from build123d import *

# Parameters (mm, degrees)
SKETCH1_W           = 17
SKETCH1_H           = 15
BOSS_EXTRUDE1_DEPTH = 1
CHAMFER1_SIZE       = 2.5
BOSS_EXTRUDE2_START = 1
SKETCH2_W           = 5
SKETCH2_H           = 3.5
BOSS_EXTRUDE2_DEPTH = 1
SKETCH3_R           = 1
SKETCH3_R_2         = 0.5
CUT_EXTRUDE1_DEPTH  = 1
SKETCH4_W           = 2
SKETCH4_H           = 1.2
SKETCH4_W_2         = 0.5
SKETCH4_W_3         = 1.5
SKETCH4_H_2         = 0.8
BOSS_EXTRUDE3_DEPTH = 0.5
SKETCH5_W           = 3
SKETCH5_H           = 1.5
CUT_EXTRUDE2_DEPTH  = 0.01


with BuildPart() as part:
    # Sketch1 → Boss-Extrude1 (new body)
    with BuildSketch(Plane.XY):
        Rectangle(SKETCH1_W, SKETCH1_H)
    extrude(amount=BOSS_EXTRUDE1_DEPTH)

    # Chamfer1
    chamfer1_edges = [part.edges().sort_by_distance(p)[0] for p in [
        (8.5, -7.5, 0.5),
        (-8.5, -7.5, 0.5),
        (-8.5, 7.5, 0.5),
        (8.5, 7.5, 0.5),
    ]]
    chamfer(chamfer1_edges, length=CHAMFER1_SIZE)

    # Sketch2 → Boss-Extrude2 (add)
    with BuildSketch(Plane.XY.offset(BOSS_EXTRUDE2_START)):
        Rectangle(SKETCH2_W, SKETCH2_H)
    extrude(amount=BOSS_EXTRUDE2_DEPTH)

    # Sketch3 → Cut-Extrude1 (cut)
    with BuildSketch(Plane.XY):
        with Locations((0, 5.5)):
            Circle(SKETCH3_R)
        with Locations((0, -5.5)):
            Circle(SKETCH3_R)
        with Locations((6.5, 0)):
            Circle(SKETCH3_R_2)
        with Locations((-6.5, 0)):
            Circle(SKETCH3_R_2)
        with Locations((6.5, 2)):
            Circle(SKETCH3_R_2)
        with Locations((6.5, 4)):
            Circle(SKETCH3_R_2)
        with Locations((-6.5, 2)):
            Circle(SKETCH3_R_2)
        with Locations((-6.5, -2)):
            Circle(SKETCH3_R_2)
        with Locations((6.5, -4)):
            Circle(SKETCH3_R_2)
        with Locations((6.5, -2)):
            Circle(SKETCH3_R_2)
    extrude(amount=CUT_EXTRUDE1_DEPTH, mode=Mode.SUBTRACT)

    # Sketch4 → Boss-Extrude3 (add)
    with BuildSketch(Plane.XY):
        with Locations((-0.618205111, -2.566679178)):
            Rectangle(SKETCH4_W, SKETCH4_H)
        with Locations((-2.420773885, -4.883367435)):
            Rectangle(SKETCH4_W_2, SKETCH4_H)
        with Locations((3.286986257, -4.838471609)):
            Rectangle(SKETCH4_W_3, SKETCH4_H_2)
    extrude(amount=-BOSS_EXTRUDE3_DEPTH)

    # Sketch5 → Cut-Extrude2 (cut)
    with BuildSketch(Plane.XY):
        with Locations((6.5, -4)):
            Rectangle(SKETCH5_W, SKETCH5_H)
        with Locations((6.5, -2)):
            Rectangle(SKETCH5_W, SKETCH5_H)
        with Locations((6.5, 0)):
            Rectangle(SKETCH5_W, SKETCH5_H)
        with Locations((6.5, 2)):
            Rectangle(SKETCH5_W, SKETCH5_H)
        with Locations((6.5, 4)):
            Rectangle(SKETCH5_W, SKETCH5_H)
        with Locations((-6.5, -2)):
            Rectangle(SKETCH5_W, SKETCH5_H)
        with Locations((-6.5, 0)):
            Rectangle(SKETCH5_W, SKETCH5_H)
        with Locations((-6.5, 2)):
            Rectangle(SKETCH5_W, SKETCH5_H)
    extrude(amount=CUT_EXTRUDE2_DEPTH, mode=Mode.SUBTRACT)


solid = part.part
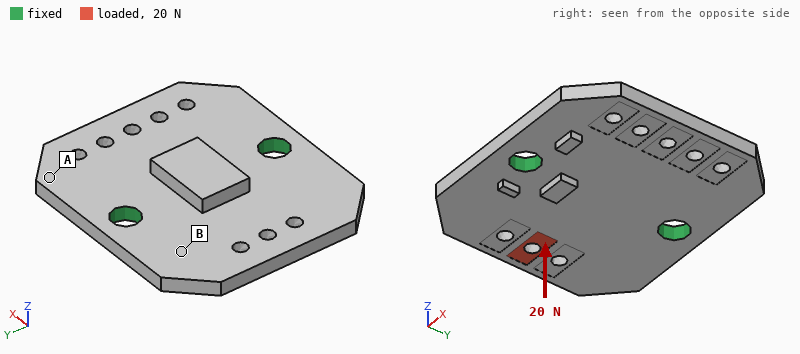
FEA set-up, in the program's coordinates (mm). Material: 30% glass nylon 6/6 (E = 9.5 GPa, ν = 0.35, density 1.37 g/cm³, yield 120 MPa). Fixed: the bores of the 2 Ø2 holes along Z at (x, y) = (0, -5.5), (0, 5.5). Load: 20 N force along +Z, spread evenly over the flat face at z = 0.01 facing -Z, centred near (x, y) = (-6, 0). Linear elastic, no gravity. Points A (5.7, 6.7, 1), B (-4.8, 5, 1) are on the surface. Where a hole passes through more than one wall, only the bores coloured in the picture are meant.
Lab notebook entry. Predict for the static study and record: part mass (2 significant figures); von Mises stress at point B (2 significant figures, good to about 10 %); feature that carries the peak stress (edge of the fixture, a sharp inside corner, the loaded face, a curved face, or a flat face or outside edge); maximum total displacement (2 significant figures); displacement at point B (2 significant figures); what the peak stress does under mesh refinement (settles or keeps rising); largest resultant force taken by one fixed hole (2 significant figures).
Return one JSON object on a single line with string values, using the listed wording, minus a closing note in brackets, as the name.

{"part mass": "0.34 g", "von Mises stress at point B": "16 MPa", "feature that carries the peak stress": "edge of the fixture", "maximum total displacement": "0.23 mm", "displacement at point B": "0.067 mm", "what the peak stress does under mesh refinement": "keeps rising", "largest resultant force taken by one fixed hole": "12 N"}
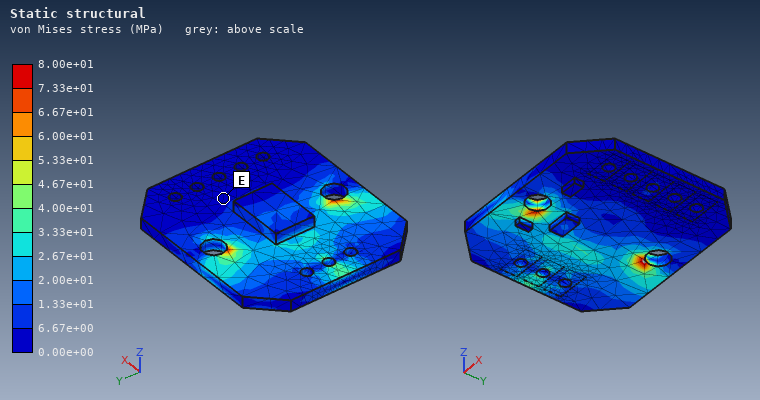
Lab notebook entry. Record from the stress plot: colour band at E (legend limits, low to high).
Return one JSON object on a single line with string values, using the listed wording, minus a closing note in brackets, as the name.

{"colour band at E": "0.00e+00 to 6.67e+00 MPa"}
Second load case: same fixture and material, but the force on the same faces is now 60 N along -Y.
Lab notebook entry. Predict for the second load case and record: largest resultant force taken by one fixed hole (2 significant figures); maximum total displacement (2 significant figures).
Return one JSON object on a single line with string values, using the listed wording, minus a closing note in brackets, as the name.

{"largest resultant force taken by one fixed hole": "44 N", "maximum total displacement": "35 µm"}
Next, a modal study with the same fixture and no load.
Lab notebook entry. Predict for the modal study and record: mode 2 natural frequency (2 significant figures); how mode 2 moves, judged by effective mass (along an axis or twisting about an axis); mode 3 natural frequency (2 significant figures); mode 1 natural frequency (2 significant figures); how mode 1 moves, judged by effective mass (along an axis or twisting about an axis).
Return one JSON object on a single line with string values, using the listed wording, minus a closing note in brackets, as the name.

{"mode 2 natural frequency": "8500 Hz", "how mode 2 moves, judged by effective mass": "along Z", "mode 3 natural frequency": "13 kHz", "mode 1 natural frequency": "6500 Hz", "how mode 1 moves, judged by effective mass": "twisting about Y"}
